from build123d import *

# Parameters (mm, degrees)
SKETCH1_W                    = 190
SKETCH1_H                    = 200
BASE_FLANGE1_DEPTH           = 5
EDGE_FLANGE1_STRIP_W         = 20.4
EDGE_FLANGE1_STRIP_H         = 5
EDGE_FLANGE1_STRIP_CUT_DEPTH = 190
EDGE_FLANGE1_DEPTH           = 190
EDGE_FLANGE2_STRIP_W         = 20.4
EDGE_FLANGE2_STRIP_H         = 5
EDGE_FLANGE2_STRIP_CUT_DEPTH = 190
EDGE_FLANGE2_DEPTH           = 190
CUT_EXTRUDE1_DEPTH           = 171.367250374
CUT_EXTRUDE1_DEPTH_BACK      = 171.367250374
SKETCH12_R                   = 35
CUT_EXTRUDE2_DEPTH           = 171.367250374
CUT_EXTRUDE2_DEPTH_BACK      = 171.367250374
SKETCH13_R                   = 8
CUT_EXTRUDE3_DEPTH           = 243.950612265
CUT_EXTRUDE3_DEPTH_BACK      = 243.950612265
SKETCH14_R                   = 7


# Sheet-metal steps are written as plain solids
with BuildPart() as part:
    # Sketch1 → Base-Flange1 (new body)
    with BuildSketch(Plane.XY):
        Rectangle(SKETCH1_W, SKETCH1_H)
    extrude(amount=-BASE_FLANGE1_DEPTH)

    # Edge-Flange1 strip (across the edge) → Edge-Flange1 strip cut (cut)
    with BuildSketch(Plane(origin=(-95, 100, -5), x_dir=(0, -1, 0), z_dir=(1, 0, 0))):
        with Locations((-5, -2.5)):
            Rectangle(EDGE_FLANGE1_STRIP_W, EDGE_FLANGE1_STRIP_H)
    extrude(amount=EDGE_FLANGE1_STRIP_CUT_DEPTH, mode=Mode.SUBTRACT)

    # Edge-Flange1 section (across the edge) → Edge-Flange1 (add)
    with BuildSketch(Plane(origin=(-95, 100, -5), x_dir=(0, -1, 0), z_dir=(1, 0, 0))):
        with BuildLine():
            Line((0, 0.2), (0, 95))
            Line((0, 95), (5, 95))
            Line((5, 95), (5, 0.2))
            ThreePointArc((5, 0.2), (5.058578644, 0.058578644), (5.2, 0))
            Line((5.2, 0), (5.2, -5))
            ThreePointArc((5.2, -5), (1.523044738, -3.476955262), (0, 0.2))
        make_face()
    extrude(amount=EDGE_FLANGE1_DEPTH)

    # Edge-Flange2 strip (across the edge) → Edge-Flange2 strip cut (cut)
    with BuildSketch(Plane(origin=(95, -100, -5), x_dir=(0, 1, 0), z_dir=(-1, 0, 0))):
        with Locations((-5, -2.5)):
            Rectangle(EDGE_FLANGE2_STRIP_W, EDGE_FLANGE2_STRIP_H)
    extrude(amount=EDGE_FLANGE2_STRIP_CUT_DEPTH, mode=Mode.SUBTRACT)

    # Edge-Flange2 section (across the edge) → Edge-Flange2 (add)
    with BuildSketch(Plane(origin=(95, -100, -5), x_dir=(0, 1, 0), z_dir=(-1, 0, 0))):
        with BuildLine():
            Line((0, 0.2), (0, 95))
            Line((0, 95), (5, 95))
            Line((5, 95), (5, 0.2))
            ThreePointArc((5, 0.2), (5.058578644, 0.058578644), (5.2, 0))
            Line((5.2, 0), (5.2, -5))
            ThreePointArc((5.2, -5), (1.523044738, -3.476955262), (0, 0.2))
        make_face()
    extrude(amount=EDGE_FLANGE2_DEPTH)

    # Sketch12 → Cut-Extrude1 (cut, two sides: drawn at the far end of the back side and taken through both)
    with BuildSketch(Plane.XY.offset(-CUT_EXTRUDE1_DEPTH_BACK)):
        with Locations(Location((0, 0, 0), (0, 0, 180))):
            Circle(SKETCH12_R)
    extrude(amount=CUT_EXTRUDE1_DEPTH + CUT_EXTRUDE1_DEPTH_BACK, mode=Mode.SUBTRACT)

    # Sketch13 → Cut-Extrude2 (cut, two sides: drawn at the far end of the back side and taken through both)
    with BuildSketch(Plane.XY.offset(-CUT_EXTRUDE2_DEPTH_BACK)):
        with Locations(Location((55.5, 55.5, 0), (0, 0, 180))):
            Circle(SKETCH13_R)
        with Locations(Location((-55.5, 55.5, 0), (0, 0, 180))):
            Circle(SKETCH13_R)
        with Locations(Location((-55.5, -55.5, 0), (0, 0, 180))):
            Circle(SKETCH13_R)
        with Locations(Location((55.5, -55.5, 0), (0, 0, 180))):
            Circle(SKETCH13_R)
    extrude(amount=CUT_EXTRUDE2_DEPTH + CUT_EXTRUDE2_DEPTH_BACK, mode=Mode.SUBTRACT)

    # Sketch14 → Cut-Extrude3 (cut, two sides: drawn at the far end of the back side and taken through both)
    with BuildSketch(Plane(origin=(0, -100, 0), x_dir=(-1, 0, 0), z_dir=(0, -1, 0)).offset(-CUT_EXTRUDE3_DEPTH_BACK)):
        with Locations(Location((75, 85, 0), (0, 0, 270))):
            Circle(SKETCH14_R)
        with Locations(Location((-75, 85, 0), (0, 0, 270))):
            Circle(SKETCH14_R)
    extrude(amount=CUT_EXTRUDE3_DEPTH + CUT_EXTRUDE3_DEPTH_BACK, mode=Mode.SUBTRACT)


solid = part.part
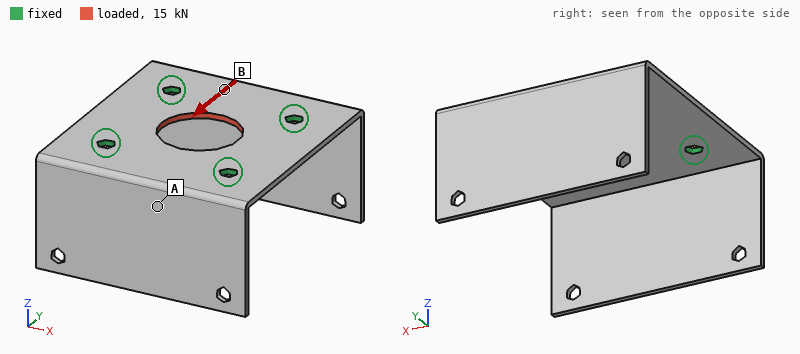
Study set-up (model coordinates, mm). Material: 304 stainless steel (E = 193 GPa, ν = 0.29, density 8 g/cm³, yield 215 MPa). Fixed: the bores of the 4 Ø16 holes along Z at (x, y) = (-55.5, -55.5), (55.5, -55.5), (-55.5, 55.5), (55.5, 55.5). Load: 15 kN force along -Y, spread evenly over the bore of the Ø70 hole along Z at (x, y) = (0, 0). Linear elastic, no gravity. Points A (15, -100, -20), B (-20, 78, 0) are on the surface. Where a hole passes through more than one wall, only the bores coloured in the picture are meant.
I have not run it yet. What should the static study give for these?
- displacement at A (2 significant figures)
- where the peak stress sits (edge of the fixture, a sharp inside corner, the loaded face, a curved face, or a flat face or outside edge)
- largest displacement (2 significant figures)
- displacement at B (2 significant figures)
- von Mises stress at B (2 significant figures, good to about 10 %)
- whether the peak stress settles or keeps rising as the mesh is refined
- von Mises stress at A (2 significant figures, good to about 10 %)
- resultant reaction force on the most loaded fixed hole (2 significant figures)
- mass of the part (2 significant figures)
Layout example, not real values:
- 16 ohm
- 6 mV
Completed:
- 3.1 µm
- edge of the fixture
- 5.8 µm
- 3.2 µm
- 8.0 MPa
- keeps rising
- 3.1 MPa
- 3.8 kN
- 2.7 kg
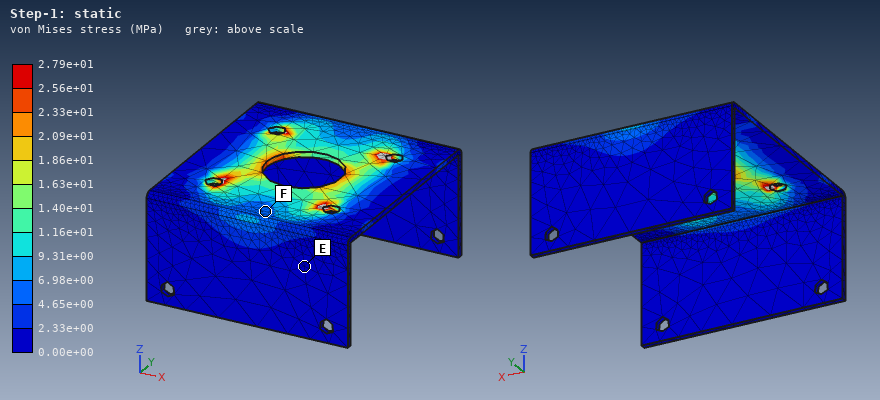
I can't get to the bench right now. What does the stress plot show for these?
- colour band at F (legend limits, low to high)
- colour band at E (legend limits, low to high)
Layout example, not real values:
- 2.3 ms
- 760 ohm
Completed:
- 4.65e+00 to 6.98e+00 MPa
- 0.00e+00 to 2.33e+00 MPa
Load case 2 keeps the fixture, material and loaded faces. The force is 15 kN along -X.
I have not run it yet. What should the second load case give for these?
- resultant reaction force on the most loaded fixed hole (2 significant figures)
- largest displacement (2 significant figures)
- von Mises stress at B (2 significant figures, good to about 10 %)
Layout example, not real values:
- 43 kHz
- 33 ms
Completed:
- 3.9 kN
- 6.2 µm
- 2.5 MPa
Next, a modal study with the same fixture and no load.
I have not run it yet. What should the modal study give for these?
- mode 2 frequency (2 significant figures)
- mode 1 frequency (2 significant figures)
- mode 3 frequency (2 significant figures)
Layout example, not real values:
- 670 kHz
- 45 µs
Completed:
- 260 Hz
- 260 Hz
- 500 Hz
